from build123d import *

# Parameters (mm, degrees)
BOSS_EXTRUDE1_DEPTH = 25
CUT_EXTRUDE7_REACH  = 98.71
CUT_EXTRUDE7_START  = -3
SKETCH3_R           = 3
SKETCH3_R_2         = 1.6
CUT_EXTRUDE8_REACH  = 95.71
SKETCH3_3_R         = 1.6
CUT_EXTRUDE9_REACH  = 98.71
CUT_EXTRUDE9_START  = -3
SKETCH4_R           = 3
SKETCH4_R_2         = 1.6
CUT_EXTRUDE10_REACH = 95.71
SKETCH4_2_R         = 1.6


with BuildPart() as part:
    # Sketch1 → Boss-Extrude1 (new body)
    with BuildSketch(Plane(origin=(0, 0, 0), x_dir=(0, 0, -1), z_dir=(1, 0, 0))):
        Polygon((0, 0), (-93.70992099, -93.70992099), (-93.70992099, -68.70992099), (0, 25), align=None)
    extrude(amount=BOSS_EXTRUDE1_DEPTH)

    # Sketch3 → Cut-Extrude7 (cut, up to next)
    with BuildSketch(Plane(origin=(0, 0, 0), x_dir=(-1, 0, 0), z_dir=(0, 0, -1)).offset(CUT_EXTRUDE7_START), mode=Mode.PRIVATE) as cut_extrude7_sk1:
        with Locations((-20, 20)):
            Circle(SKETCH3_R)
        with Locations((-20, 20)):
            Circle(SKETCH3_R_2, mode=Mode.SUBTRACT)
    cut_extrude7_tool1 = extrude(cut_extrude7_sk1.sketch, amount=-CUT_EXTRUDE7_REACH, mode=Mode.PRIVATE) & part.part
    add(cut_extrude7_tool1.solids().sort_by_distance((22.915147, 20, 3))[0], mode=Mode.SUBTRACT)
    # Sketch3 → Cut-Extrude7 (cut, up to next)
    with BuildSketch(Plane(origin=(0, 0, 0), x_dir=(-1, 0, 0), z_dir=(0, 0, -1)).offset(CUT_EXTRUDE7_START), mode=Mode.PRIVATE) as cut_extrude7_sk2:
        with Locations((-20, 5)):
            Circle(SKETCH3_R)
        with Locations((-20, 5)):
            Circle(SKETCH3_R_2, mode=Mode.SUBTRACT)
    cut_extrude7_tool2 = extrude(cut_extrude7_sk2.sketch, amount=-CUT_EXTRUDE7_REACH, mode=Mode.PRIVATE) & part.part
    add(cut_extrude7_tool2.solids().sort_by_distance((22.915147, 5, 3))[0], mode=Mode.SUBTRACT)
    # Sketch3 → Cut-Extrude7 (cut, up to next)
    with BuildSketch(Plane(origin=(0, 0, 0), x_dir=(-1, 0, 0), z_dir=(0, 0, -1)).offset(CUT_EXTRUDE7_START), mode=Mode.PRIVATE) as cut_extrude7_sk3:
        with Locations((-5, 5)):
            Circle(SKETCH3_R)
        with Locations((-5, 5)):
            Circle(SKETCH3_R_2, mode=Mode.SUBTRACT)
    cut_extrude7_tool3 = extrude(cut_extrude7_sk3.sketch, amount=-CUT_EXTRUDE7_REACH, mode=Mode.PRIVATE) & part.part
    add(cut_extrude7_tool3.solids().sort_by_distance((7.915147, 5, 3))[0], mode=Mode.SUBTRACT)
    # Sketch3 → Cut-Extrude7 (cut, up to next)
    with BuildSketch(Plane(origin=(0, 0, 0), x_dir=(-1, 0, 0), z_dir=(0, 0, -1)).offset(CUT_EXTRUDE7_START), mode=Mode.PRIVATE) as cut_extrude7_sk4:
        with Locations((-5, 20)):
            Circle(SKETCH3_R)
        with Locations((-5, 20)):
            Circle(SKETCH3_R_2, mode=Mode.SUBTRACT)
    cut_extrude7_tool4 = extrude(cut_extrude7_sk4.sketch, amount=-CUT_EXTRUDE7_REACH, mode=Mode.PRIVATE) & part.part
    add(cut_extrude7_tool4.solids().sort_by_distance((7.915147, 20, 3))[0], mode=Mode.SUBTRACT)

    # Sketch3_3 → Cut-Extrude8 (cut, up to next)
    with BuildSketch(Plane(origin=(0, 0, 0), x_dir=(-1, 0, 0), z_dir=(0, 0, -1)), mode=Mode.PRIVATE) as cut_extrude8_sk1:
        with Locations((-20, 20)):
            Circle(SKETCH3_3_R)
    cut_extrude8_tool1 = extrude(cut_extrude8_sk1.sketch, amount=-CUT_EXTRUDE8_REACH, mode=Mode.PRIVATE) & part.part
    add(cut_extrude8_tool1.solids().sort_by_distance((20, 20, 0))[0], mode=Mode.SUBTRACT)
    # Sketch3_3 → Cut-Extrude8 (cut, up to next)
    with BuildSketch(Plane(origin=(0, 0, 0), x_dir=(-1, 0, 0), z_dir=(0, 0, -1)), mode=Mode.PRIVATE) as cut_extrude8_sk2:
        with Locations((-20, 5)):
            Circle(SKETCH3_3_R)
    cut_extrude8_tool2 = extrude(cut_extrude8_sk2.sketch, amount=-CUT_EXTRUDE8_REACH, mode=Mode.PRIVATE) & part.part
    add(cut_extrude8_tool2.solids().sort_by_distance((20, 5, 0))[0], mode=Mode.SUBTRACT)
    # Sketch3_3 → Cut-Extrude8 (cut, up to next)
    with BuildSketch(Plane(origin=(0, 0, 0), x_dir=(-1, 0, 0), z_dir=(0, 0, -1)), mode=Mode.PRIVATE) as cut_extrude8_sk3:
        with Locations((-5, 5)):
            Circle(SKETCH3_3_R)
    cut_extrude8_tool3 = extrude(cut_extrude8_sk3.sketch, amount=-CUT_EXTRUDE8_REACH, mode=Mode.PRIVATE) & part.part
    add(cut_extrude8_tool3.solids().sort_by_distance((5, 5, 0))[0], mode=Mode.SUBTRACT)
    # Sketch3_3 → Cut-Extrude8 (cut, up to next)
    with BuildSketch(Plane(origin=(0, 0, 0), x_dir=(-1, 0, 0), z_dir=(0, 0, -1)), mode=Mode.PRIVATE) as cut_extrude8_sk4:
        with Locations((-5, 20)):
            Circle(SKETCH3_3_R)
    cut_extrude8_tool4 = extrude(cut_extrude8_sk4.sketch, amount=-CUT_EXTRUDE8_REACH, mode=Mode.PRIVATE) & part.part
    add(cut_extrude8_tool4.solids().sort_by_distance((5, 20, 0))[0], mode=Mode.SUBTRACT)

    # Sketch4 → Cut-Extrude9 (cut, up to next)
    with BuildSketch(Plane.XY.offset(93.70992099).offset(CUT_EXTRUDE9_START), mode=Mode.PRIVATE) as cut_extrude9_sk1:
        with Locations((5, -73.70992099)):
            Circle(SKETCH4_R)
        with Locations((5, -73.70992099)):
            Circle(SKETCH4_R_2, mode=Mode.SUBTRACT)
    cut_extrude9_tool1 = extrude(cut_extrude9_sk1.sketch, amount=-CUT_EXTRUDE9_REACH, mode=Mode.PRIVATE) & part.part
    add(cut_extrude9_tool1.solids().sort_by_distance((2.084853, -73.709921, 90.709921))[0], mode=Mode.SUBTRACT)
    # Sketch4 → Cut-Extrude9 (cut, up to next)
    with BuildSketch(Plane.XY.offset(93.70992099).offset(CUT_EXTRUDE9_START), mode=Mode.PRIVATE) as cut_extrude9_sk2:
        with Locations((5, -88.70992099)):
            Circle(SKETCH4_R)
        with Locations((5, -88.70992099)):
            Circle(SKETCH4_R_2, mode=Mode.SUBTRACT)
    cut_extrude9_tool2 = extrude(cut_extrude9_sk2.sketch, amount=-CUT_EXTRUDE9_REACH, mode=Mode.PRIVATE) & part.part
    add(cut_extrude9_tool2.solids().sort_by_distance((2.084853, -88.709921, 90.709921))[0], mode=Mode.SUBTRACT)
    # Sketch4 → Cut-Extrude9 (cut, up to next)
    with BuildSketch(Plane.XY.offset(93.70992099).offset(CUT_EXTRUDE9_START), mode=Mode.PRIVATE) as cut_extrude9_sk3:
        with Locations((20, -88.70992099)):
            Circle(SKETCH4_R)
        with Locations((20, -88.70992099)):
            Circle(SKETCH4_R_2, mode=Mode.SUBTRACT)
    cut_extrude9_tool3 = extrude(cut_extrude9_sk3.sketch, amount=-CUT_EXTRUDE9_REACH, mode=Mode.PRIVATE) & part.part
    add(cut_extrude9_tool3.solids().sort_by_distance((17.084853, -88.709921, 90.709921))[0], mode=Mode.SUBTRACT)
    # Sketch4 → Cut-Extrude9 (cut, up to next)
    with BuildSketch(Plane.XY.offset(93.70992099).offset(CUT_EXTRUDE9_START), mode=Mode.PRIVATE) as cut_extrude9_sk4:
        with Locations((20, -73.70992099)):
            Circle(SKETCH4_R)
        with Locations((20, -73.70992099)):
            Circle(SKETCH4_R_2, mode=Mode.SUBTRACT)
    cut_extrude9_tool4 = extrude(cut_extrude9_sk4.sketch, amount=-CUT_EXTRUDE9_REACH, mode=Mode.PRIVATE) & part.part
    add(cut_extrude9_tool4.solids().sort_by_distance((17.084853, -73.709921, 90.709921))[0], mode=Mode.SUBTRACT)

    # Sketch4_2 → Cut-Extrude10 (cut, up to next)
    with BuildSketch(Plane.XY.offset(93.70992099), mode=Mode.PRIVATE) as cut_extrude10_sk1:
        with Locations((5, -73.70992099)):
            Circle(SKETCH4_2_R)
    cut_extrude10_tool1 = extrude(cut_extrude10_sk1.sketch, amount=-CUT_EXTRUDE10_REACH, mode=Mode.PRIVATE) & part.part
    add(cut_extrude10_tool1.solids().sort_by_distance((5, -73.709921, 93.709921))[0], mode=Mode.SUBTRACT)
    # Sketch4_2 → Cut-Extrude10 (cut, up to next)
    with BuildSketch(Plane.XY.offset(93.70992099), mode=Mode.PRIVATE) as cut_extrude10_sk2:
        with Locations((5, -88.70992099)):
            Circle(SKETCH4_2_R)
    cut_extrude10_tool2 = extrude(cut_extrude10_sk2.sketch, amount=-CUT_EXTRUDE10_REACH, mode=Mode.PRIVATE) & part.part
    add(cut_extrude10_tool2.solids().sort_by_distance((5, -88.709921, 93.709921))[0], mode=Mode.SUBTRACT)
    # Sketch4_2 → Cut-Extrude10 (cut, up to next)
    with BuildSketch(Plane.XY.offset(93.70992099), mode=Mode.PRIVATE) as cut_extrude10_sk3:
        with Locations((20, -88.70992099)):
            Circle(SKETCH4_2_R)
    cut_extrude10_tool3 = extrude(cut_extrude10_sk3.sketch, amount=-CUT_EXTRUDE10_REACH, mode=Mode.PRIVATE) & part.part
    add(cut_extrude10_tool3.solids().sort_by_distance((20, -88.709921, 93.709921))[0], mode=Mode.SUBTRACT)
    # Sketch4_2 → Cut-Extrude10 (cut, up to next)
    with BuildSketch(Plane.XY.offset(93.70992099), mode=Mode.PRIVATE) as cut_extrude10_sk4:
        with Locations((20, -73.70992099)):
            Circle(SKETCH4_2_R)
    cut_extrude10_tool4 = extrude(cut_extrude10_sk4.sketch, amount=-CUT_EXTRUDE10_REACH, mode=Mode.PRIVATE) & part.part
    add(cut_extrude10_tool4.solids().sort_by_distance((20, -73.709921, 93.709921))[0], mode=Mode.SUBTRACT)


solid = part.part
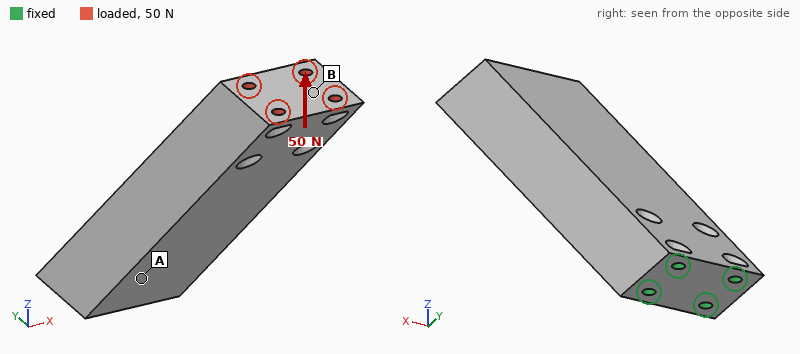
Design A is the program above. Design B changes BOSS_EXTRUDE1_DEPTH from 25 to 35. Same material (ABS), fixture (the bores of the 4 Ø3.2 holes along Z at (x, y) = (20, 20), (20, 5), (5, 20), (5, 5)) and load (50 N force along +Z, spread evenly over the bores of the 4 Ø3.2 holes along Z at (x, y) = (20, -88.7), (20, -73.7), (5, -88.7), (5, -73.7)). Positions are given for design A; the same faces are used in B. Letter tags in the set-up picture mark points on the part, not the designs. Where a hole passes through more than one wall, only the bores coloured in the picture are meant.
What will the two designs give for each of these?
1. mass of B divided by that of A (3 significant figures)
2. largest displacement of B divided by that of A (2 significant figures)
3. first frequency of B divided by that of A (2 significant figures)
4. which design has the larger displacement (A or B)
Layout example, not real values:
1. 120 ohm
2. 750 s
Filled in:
1. 1.42
2. 0.80
3. 0.93
4. A
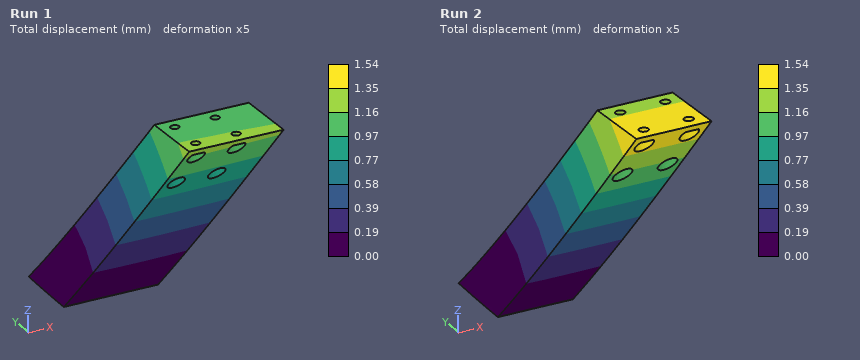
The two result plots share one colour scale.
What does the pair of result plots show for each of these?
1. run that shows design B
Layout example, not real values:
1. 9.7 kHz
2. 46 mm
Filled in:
1. Run 1
